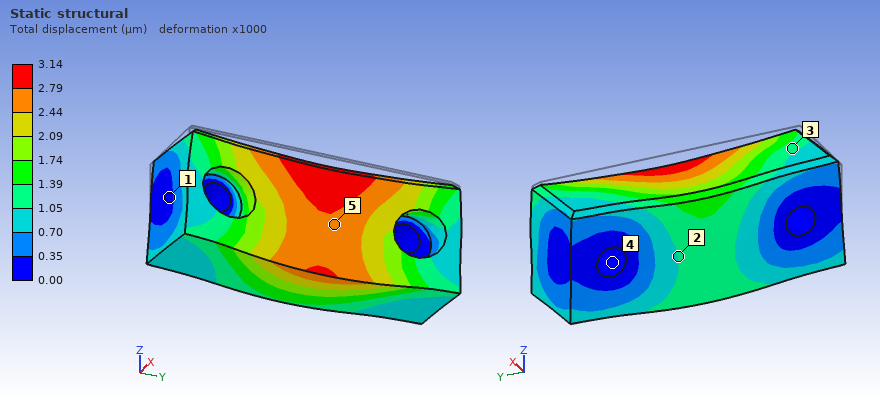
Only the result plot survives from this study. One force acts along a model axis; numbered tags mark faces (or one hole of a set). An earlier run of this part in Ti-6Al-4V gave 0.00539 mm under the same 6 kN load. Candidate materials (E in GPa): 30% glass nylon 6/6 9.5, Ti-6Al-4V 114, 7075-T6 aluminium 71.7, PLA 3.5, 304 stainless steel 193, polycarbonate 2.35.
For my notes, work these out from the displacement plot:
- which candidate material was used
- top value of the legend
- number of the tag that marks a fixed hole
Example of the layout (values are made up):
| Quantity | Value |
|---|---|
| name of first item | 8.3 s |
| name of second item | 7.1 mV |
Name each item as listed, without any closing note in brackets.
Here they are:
| Quantity | Value |
|---|---|
| which candidate material was used | 304 stainless steel |
| top value of the legend | 3.14 µm |
| number of the tag that marks a fixed hole | 4 |
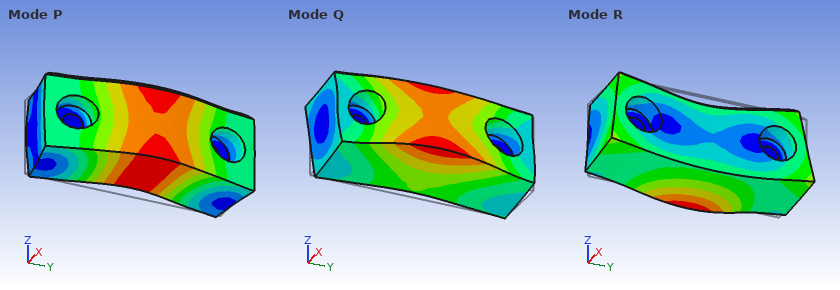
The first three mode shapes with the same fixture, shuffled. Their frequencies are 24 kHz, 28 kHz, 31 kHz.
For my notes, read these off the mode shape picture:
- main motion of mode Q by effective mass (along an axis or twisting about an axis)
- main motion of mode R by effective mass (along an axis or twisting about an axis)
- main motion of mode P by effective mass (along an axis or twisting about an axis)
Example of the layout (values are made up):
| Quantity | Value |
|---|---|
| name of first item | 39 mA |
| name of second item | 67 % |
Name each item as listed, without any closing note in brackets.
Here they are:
| Quantity | Value |
|---|---|
| main motion of mode Q by effective mass | along Z |
| main motion of mode R by effective mass | along Z |
| main motion of mode P by effective mass | along X |
